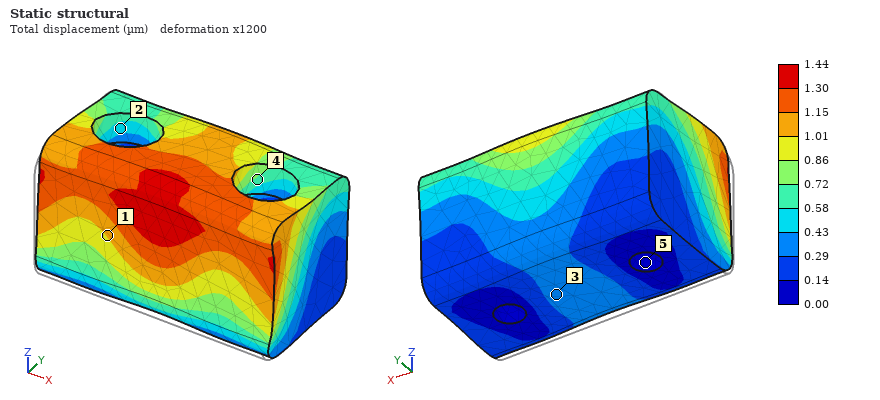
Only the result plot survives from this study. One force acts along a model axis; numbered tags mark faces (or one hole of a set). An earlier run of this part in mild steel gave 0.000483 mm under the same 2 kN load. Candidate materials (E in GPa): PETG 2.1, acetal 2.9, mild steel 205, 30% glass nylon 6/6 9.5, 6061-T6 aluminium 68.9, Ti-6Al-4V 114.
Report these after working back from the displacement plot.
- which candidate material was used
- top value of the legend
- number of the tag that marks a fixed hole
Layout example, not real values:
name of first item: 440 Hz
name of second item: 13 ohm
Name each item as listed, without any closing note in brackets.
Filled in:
which candidate material was used: 6061-T6 aluminium
top value of the legend: 1.44 µm
number of the tag that marks a fixed hole: 5
